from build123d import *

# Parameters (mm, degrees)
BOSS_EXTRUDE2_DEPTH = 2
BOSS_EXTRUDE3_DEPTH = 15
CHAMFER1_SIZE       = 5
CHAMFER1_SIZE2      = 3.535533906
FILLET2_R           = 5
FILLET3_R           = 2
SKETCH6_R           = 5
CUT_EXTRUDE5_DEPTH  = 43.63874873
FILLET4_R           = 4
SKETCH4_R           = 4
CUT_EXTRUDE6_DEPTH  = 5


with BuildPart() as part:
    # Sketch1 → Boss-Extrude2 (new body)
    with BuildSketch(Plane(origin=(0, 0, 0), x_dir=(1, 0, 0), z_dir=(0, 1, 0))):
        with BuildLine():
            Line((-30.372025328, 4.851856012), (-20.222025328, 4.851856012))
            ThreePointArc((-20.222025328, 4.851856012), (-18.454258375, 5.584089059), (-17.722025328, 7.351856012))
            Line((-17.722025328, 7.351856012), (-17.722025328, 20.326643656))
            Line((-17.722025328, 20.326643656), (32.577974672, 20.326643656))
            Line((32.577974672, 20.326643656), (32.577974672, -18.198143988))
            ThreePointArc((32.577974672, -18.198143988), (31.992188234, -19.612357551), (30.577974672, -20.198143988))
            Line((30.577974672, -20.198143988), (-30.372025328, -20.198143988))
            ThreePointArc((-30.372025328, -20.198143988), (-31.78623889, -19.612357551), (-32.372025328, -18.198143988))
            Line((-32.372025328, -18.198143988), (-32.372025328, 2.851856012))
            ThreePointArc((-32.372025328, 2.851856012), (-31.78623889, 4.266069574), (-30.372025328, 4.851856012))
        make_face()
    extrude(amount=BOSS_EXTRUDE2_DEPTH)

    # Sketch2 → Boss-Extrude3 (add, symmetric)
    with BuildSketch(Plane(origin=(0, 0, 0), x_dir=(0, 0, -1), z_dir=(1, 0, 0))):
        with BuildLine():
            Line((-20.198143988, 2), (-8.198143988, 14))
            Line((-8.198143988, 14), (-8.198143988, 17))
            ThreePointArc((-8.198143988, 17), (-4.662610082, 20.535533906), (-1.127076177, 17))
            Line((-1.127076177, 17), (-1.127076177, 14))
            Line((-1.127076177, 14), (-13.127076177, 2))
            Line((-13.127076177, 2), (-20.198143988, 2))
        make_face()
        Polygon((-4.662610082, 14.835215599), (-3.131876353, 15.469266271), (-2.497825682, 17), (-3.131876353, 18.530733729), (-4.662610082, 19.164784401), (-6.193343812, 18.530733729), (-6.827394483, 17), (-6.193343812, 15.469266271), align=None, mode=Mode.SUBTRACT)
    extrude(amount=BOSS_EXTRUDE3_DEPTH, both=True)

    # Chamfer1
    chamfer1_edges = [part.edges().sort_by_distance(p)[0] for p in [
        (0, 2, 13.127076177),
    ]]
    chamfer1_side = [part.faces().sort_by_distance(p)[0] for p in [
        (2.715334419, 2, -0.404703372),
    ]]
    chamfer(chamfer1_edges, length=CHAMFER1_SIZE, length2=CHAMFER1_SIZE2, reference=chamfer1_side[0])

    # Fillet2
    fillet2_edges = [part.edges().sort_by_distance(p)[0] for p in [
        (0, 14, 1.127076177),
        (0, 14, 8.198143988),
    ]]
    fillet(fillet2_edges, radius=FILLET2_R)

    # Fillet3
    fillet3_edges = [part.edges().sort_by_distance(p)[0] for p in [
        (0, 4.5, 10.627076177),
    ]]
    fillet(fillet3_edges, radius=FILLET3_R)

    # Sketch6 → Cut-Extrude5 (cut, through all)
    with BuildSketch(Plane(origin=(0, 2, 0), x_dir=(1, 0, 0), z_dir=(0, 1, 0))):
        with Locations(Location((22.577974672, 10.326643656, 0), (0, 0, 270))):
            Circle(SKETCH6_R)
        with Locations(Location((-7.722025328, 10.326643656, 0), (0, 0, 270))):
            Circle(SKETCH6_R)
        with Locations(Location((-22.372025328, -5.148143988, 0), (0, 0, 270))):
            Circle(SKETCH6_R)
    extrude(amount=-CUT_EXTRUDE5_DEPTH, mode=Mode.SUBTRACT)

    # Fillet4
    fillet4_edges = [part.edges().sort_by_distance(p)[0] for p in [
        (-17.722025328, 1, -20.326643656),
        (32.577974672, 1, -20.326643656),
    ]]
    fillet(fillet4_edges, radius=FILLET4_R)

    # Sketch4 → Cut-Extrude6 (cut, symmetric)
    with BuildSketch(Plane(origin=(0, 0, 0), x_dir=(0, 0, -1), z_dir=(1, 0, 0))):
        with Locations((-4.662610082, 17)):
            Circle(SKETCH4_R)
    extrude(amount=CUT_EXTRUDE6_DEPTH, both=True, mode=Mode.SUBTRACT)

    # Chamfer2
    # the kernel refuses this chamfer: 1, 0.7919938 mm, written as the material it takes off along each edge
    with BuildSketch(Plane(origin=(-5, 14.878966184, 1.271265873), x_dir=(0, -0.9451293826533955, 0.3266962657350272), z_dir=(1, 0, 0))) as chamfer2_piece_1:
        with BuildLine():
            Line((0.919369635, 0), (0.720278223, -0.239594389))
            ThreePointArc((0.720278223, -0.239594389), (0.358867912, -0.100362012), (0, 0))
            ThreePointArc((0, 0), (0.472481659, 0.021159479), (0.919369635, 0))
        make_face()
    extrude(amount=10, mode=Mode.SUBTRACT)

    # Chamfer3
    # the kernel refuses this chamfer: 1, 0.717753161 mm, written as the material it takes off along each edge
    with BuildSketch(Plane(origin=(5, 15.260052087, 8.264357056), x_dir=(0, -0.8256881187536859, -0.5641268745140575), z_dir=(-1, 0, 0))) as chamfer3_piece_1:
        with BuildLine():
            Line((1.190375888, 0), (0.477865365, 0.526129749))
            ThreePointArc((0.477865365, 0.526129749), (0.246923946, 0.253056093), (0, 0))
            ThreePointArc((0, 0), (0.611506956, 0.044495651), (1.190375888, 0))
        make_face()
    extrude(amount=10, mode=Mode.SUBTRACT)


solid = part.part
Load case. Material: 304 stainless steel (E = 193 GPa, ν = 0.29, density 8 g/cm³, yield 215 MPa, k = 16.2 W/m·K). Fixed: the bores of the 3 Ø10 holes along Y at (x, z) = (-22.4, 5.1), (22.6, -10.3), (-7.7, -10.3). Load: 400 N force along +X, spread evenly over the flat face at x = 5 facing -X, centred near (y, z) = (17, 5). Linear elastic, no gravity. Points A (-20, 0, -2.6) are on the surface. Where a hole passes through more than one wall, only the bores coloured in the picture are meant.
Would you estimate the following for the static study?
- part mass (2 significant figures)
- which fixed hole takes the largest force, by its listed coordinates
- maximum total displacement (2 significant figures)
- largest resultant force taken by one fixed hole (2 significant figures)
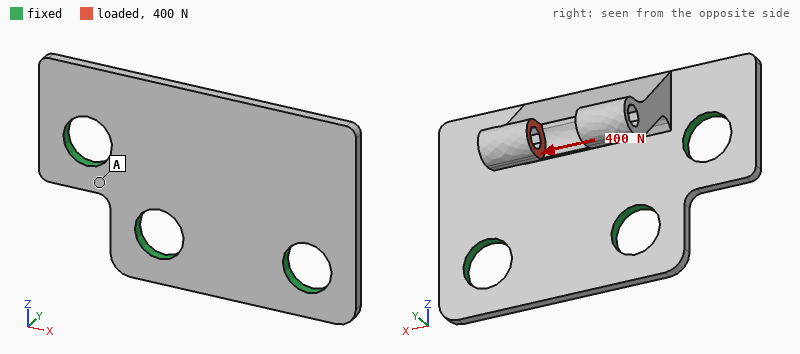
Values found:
61 g
(-22.4, 5.1)
70 µm
310 N
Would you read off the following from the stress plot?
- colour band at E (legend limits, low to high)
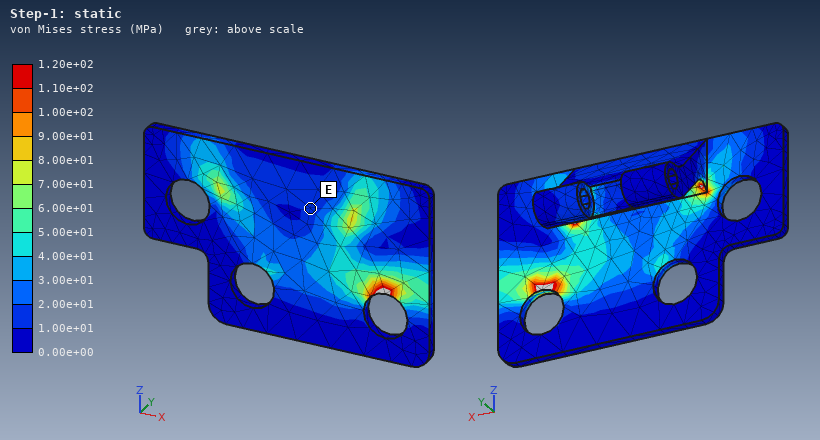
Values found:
1.00e+01 to 2.00e+01 MPa
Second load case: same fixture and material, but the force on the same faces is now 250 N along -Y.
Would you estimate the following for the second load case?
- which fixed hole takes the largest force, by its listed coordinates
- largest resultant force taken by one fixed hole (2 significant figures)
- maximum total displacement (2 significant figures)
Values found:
(22.6, -10.3)
120 N
34 µm
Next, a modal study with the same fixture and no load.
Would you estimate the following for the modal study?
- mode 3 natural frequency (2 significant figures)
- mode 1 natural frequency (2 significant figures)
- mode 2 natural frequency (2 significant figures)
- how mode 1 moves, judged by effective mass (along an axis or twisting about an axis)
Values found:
6900 Hz
2000 Hz
4300 Hz
along Y
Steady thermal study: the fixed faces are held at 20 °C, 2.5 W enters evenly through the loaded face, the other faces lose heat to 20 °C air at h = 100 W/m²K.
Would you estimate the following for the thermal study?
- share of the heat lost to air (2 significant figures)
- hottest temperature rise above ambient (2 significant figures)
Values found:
87 %
40 K
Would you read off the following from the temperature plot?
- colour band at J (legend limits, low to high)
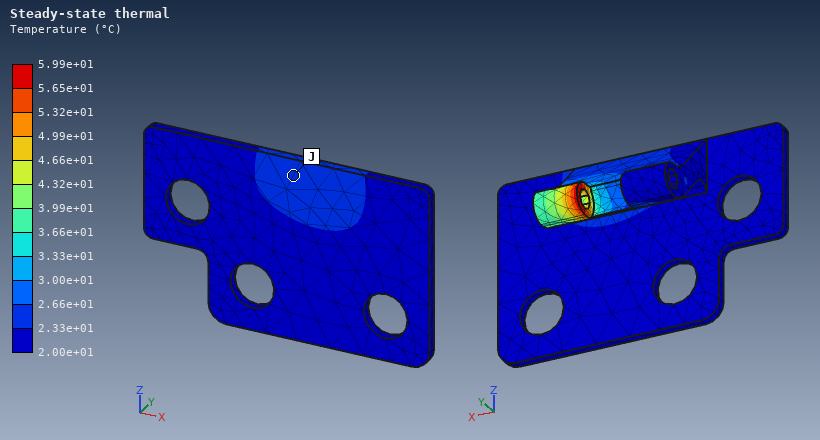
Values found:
2.33e+01 to 2.66e+01 °C
